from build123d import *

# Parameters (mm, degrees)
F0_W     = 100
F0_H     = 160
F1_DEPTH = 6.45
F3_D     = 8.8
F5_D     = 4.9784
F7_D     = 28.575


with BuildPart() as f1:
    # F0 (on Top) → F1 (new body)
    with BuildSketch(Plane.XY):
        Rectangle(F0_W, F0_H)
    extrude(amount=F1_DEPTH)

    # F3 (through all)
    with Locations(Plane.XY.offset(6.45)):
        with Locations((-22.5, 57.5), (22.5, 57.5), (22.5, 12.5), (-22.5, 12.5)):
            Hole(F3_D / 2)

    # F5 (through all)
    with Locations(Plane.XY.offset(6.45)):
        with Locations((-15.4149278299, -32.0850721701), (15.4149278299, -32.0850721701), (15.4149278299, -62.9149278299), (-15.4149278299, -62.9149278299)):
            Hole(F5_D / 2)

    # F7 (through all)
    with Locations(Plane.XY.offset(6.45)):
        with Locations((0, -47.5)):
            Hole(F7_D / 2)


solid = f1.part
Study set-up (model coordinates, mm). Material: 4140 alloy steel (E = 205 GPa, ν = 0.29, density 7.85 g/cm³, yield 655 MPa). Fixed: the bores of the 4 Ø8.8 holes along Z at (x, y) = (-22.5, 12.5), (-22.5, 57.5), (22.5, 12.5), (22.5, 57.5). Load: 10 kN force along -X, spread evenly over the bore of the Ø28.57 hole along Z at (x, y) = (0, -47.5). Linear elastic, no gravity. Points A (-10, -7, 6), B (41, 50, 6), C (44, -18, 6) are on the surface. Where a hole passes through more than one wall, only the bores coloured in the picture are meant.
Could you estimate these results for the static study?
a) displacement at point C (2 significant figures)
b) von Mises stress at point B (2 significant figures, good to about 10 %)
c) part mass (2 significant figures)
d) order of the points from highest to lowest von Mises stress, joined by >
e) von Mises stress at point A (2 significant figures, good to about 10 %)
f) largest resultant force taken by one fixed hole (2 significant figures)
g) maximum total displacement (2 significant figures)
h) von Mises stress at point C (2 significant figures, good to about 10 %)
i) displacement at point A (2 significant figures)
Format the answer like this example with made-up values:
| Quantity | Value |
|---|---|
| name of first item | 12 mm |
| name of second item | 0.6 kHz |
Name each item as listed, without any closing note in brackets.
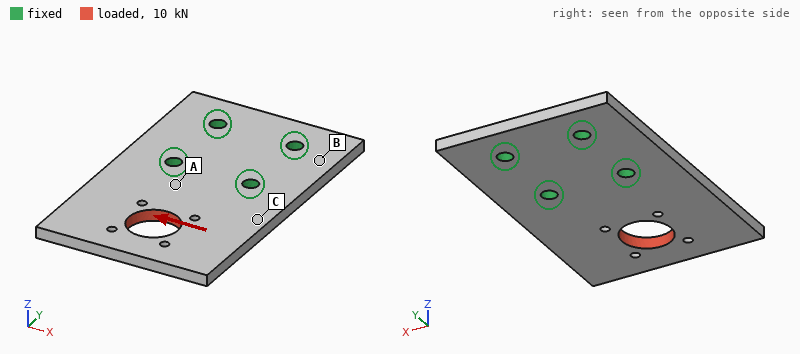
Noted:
| Quantity | Value |
|---|---|
| displacement at point C | 17 µm |
| von Mises stress at point B | 12 MPa |
| part mass | 760 g |
| order of the points from highest to lowest von Mises stress, joined by > | A > C > B |
| von Mises stress at point A | 49 MPa |
| largest resultant force taken by one fixed hole | 9.5 kN |
| maximum total displacement | 47 µm |
| von Mises stress at point C | 27 MPa |
| displacement at point A | 7.5 µm |
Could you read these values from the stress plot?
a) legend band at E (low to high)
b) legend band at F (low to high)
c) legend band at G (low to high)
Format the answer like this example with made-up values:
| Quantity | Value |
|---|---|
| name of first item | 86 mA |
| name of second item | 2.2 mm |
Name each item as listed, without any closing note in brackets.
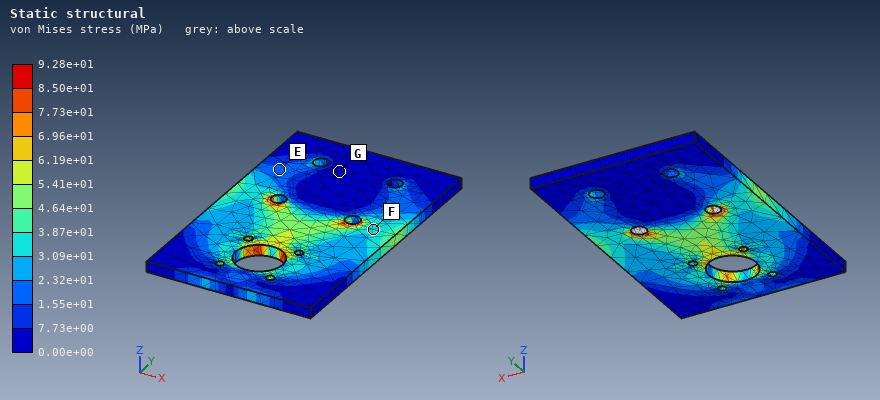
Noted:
| Quantity | Value |
|---|---|
| legend band at E | 1.55e+01 to 2.32e+01 MPa |
| legend band at F | 3.09e+01 to 3.87e+01 MPa |
| legend band at G | 0.00e+00 to 7.73e+00 MPa |
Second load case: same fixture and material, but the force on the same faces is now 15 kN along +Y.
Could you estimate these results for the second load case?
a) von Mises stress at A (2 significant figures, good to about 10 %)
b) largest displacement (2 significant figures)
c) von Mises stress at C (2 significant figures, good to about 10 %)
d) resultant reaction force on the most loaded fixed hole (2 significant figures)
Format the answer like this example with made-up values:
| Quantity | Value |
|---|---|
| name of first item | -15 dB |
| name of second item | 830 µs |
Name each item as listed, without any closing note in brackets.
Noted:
| Quantity | Value |
|---|---|
| von Mises stress at A | 27 MPa |
| largest displacement | 18 µm |
| von Mises stress at C | 15 MPa |
| resultant reaction force on the most loaded fixed hole | 6.2 kN |
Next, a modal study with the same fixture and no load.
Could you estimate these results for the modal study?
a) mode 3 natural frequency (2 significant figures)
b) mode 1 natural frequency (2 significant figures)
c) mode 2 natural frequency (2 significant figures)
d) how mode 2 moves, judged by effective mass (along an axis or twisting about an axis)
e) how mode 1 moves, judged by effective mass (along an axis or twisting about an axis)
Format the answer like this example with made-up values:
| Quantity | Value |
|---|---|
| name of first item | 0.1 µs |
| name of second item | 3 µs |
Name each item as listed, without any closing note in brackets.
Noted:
| Quantity | Value |
|---|---|
| mode 3 natural frequency | 3300 Hz |
| mode 1 natural frequency | 650 Hz |
| mode 2 natural frequency | 1300 Hz |
| how mode 2 moves, judged by effective mass | twisting about Y |
| how mode 1 moves, judged by effective mass | along Z |
